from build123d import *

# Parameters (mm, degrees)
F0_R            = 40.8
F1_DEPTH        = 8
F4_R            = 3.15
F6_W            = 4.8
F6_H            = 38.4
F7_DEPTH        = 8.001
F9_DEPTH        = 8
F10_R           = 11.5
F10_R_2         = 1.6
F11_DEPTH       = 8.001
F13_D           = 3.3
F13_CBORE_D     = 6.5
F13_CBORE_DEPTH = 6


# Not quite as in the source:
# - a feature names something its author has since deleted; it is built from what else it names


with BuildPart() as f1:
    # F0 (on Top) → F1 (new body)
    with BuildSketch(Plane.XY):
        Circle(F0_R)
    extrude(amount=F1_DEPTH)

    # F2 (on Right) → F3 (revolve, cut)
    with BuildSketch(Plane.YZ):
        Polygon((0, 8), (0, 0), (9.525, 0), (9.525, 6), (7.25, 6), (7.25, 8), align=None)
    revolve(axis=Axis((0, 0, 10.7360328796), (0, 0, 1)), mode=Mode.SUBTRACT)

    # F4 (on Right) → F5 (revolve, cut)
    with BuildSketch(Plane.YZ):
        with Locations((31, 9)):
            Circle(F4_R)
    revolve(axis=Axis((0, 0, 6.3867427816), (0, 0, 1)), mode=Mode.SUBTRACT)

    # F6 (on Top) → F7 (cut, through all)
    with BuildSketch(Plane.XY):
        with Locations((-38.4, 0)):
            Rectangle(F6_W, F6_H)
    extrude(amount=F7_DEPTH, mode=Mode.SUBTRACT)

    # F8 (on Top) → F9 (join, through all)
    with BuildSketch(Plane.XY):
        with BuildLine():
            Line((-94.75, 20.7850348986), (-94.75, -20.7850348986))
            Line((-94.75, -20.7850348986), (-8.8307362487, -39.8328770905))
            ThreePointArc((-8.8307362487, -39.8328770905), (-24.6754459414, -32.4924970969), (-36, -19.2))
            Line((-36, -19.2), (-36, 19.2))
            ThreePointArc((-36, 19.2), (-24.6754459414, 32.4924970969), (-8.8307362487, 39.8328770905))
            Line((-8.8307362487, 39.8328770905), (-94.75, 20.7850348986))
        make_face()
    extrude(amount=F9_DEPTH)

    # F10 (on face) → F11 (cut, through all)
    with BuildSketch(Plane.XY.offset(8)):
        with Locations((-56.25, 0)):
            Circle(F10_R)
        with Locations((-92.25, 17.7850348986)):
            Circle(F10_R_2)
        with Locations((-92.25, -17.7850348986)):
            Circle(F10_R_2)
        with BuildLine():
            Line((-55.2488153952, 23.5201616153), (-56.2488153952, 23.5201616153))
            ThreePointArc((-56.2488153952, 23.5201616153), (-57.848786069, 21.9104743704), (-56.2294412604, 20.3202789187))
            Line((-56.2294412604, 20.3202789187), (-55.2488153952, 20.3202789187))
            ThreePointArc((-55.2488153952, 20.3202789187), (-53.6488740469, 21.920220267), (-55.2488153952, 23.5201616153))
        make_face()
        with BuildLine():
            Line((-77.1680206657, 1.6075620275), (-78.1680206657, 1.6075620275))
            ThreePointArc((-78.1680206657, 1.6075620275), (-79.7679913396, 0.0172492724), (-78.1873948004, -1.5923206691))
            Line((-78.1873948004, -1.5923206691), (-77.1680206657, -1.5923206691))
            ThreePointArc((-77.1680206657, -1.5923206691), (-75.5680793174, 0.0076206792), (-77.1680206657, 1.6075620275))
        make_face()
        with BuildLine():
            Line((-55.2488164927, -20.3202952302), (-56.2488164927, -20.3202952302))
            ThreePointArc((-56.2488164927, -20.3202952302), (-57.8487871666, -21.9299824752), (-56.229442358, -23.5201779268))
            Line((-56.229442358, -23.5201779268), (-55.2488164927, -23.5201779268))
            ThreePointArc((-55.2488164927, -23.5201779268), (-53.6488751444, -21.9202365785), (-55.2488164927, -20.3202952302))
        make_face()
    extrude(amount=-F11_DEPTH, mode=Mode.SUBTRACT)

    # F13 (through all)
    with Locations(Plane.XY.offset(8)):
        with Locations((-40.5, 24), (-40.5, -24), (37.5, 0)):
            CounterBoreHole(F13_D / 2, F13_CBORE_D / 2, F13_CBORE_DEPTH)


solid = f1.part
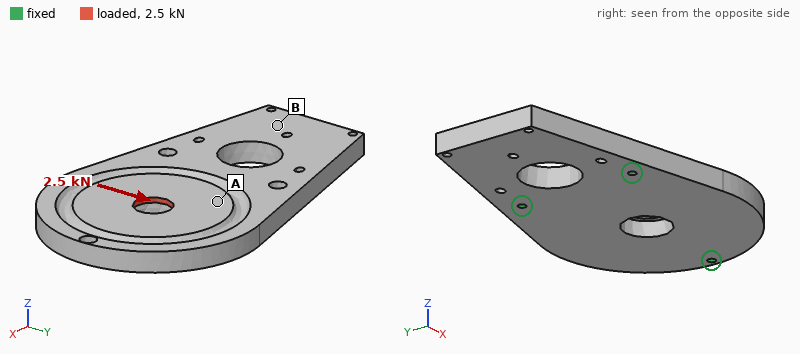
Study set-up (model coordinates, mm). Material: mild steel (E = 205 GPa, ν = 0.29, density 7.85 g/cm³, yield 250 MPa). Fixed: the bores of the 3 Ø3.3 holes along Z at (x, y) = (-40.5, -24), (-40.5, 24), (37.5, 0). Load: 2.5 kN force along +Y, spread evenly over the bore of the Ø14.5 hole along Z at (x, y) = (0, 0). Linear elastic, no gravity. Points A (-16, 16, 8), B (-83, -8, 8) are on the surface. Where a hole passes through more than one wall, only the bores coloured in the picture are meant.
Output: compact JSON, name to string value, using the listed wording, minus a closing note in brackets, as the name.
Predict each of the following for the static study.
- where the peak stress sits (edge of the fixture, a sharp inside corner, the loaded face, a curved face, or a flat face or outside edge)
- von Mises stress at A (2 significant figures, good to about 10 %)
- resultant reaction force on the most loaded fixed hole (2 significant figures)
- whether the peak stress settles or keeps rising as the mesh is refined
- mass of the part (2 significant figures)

{"where the peak stress sits": "edge of the fixture", "von Mises stress at A": "13 MPa", "resultant reaction force on the most loaded fixed hole": "1.0 kN", "whether the peak stress settles or keeps rising as the mesh is refined": "keeps rising", "mass of the part": "470 g"}
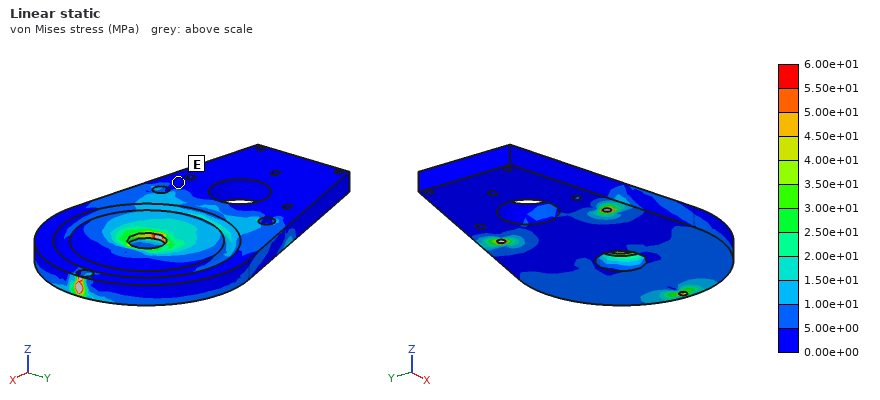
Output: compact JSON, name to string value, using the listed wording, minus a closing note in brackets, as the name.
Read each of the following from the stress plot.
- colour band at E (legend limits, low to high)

{"colour band at E": "0.00e+00 to 5.00e+00 MPa"}
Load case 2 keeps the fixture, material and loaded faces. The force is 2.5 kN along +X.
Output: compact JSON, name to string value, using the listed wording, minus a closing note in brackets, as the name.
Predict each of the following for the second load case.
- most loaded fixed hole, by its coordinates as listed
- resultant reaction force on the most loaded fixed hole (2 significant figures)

{"most loaded fixed hole, by its coordinates as listed": "(37.5, 0)", "resultant reaction force on the most loaded fixed hole": "930 N"}
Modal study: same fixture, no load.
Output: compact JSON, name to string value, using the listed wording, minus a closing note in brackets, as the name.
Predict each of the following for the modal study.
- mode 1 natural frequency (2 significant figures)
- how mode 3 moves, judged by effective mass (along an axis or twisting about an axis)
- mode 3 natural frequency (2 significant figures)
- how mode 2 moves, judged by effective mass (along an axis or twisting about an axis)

{"mode 1 natural frequency": "1500 Hz", "how mode 3 moves, judged by effective mass": "along Z", "mode 3 natural frequency": "3400 Hz", "how mode 2 moves, judged by effective mass": "twisting about X"}
